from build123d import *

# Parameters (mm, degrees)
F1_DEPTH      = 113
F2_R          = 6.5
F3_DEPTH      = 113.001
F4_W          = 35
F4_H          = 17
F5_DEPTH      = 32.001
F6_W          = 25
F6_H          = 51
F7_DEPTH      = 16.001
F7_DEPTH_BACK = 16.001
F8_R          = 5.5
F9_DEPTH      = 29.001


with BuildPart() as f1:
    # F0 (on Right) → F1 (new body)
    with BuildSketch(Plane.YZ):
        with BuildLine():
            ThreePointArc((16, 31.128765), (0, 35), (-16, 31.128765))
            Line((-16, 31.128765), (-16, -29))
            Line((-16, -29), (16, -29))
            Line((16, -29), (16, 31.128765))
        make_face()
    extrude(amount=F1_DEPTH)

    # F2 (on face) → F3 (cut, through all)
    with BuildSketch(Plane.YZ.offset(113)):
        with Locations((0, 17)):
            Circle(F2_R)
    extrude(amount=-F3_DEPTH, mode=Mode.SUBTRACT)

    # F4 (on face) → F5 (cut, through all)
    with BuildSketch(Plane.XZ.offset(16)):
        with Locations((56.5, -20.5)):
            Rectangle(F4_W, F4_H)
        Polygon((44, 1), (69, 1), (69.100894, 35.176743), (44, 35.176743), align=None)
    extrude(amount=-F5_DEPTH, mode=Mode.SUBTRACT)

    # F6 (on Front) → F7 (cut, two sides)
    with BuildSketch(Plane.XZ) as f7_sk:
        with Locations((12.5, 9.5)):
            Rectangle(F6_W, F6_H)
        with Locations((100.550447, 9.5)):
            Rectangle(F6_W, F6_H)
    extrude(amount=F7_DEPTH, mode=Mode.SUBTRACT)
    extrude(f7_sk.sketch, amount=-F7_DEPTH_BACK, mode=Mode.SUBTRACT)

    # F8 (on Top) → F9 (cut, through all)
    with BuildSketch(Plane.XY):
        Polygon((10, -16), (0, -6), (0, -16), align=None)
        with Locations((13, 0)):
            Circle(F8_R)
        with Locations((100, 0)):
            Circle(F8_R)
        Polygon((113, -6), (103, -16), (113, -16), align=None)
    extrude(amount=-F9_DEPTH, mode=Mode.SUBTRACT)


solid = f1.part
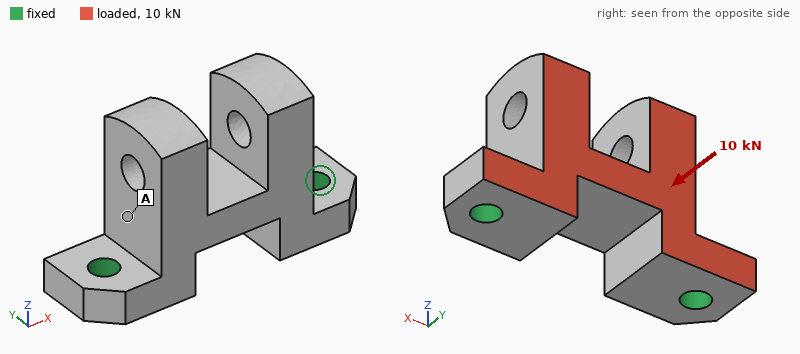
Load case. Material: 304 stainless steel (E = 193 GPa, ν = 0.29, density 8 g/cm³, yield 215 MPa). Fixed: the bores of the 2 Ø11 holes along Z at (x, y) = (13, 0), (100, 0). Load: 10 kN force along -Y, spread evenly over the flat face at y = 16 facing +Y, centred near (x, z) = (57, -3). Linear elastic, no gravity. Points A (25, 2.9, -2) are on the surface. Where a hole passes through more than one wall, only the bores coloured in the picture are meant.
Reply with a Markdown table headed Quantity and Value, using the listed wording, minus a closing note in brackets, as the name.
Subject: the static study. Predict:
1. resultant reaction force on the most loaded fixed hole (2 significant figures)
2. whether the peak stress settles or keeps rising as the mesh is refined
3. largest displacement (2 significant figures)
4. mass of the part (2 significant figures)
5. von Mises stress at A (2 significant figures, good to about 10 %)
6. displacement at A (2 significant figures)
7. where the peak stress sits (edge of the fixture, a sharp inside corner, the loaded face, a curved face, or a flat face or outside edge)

| Quantity | Value |
|---|---|
| resultant reaction force on the most loaded fixed hole | 5.0 kN |
| whether the peak stress settles or keeps rising as the mesh is refined | keeps rising |
| largest displacement | 62 µm |
| mass of the part | 750 g |
| von Mises stress at A | 19 MPa |
| displacement at A | 23 µm |
| where the peak stress sits | edge of the fixture |
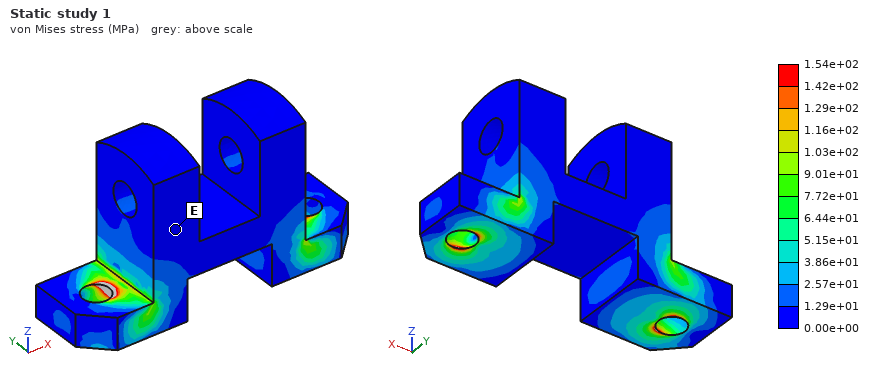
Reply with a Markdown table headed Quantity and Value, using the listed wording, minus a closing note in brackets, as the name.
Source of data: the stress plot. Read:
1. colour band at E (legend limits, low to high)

| Quantity | Value |
|---|---|
| colour band at E | 0.00e+00 to 1.29e+01 MPa |
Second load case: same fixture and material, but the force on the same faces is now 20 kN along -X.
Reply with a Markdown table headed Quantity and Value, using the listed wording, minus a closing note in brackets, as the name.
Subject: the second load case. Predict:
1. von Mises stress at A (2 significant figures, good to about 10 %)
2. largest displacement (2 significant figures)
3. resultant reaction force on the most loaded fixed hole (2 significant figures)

| Quantity | Value |
|---|---|
| von Mises stress at A | 31 MPa |
| largest displacement | 45 µm |
| resultant reaction force on the most loaded fixed hole | 12 kN |
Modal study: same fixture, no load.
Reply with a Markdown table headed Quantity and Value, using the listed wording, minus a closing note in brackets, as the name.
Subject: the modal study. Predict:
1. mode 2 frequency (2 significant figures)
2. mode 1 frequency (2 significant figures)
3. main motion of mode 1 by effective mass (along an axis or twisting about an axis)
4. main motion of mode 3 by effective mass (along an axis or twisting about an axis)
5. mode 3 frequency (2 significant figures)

| Quantity | Value |
|---|---|
| mode 2 frequency | 4600 Hz |
| mode 1 frequency | 2800 Hz |
| main motion of mode 1 by effective mass | along Y |
| main motion of mode 3 by effective mass | along X |
| mode 3 frequency | 5500 Hz |
